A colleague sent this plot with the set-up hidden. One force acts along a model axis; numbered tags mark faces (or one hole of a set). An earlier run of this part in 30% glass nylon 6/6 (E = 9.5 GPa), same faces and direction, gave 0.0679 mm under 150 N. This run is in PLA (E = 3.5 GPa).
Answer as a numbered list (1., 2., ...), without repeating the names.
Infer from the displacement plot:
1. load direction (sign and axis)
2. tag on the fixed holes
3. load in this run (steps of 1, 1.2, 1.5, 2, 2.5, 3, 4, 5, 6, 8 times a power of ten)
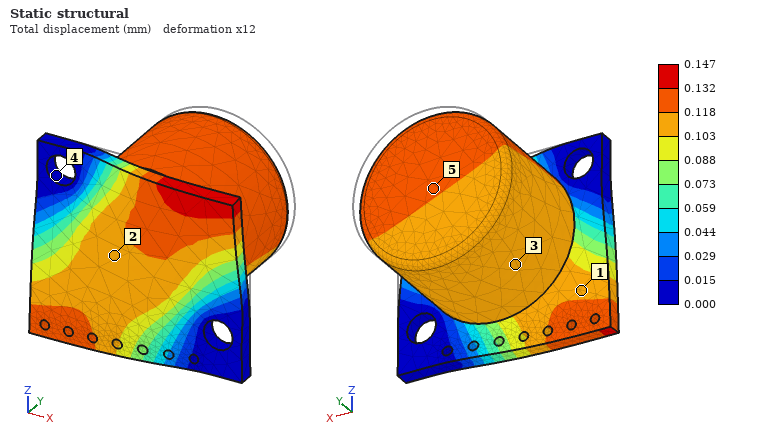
1. -Y
2. 4
3. 120 N
